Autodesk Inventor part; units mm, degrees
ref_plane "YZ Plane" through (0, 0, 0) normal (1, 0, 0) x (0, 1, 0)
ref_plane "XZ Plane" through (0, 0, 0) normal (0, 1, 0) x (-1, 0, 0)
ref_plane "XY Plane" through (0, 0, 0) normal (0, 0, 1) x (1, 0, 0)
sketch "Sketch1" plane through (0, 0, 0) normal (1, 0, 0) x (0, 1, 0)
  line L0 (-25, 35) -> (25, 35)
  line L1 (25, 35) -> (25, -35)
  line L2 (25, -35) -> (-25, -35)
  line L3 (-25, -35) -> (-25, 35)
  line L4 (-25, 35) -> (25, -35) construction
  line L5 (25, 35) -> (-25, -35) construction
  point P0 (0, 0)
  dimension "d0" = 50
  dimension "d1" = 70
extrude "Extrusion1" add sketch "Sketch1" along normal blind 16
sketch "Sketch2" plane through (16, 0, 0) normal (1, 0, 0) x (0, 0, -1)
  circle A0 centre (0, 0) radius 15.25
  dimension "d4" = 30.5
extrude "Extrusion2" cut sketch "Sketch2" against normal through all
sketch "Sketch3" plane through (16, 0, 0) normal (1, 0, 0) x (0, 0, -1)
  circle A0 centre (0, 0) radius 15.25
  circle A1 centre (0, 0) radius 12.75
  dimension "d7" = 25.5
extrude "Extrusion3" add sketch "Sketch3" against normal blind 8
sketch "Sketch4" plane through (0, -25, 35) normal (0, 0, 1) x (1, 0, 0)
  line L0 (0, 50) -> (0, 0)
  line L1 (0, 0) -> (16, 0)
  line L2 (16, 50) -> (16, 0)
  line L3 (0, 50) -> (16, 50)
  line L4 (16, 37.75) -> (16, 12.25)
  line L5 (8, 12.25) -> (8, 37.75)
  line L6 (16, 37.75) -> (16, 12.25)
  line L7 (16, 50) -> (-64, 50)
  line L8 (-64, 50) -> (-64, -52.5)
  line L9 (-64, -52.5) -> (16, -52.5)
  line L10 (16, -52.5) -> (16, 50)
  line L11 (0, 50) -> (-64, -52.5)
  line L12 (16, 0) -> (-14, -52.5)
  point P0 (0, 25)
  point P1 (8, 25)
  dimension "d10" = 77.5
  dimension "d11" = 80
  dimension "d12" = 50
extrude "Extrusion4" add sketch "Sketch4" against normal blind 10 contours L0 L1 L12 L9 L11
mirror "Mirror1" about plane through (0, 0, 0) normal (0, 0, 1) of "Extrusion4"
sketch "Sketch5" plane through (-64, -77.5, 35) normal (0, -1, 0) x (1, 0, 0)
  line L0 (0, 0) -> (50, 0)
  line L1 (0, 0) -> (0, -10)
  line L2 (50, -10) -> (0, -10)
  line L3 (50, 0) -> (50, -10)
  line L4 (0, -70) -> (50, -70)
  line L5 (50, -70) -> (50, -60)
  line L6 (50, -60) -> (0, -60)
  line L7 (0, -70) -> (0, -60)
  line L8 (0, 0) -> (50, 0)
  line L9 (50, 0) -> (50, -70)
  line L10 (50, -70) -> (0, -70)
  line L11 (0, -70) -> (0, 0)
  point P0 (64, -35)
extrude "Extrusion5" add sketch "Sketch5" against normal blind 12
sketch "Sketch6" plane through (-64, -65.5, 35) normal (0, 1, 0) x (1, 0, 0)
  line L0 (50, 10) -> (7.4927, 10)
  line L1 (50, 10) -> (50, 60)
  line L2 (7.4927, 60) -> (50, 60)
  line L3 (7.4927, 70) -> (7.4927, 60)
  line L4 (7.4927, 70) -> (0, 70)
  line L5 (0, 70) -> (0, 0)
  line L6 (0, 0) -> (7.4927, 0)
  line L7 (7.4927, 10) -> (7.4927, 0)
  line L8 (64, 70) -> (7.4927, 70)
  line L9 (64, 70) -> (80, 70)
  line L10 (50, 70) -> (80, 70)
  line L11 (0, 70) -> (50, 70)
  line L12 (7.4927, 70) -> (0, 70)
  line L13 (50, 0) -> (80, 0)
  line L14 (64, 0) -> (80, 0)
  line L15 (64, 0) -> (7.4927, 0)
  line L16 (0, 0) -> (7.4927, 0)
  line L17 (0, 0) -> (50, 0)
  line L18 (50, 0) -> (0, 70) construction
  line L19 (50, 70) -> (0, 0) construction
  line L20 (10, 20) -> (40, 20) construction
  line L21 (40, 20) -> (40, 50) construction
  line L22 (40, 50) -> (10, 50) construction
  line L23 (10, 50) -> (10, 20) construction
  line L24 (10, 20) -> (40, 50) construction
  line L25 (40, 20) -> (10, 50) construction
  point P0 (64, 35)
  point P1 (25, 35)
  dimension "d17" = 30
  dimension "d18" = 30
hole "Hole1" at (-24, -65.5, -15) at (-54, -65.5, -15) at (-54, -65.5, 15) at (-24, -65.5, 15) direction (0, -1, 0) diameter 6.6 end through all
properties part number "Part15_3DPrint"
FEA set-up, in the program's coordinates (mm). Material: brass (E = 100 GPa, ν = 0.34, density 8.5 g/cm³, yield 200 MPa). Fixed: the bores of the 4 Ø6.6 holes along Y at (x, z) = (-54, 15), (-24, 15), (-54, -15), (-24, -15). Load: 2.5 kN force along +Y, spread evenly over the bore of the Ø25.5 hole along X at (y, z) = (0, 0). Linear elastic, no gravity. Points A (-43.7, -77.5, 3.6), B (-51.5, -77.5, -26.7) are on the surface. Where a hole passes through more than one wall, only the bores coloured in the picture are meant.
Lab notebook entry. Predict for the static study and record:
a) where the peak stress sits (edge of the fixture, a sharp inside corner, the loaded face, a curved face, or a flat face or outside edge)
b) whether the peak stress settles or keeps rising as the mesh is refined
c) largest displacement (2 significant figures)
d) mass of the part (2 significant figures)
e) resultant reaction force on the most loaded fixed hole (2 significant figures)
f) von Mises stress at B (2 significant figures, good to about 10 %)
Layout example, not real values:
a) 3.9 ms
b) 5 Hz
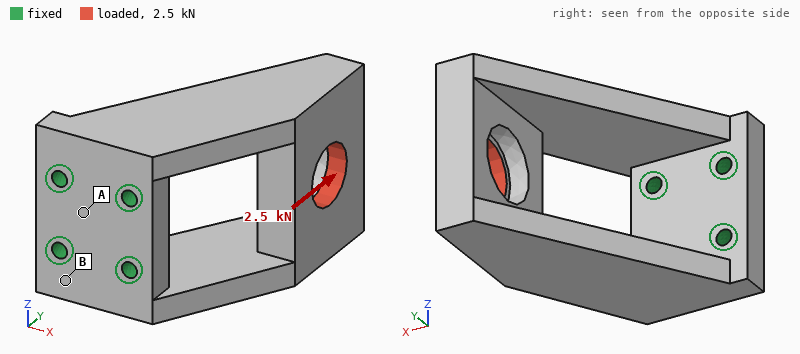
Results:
a) edge of the fixture
b) keeps rising
c) 77 µm
d) 1.2 kg
e) 2.4 kN
f) 10 MPa
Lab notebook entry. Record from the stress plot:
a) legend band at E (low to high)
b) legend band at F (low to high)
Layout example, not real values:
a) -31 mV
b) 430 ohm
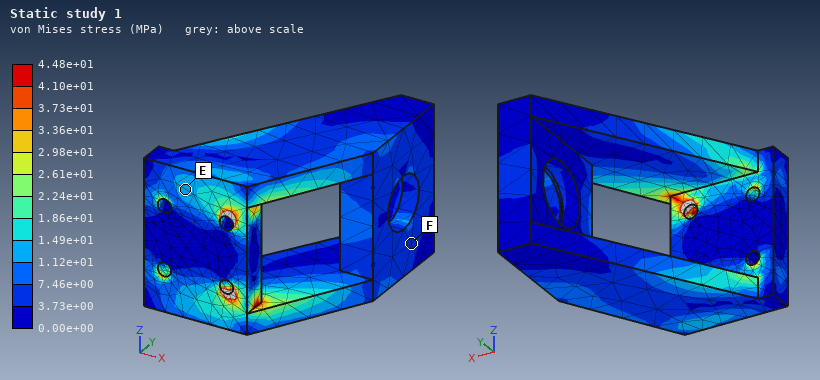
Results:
a) 1.12e+01 to 1.49e+01 MPa
b) 3.73e+00 to 7.46e+00 MPa
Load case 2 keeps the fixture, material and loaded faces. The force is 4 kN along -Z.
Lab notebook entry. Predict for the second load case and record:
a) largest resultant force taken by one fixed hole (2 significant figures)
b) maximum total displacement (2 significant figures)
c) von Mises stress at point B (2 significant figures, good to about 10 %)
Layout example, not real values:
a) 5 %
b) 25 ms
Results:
a) 4.2 kN
b) 0.29 mm
c) 37 MPa
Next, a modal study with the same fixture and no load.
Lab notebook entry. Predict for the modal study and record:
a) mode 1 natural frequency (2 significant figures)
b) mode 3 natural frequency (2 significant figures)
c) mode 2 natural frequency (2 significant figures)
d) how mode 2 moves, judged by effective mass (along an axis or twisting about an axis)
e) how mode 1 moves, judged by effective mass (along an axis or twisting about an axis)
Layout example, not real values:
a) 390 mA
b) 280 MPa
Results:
a) 830 Hz
b) 2000 Hz
c) 1100 Hz
d) along X
e) along Z
